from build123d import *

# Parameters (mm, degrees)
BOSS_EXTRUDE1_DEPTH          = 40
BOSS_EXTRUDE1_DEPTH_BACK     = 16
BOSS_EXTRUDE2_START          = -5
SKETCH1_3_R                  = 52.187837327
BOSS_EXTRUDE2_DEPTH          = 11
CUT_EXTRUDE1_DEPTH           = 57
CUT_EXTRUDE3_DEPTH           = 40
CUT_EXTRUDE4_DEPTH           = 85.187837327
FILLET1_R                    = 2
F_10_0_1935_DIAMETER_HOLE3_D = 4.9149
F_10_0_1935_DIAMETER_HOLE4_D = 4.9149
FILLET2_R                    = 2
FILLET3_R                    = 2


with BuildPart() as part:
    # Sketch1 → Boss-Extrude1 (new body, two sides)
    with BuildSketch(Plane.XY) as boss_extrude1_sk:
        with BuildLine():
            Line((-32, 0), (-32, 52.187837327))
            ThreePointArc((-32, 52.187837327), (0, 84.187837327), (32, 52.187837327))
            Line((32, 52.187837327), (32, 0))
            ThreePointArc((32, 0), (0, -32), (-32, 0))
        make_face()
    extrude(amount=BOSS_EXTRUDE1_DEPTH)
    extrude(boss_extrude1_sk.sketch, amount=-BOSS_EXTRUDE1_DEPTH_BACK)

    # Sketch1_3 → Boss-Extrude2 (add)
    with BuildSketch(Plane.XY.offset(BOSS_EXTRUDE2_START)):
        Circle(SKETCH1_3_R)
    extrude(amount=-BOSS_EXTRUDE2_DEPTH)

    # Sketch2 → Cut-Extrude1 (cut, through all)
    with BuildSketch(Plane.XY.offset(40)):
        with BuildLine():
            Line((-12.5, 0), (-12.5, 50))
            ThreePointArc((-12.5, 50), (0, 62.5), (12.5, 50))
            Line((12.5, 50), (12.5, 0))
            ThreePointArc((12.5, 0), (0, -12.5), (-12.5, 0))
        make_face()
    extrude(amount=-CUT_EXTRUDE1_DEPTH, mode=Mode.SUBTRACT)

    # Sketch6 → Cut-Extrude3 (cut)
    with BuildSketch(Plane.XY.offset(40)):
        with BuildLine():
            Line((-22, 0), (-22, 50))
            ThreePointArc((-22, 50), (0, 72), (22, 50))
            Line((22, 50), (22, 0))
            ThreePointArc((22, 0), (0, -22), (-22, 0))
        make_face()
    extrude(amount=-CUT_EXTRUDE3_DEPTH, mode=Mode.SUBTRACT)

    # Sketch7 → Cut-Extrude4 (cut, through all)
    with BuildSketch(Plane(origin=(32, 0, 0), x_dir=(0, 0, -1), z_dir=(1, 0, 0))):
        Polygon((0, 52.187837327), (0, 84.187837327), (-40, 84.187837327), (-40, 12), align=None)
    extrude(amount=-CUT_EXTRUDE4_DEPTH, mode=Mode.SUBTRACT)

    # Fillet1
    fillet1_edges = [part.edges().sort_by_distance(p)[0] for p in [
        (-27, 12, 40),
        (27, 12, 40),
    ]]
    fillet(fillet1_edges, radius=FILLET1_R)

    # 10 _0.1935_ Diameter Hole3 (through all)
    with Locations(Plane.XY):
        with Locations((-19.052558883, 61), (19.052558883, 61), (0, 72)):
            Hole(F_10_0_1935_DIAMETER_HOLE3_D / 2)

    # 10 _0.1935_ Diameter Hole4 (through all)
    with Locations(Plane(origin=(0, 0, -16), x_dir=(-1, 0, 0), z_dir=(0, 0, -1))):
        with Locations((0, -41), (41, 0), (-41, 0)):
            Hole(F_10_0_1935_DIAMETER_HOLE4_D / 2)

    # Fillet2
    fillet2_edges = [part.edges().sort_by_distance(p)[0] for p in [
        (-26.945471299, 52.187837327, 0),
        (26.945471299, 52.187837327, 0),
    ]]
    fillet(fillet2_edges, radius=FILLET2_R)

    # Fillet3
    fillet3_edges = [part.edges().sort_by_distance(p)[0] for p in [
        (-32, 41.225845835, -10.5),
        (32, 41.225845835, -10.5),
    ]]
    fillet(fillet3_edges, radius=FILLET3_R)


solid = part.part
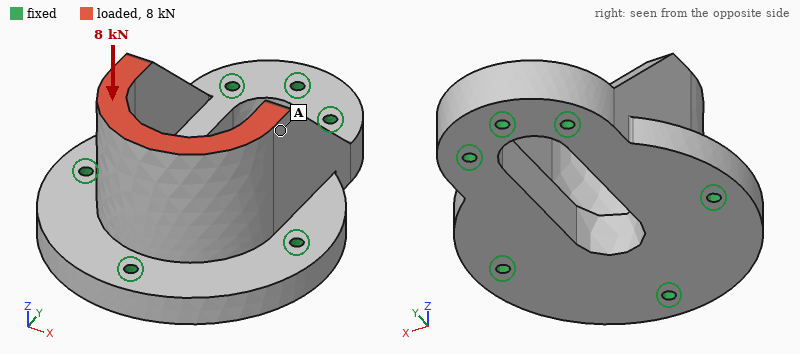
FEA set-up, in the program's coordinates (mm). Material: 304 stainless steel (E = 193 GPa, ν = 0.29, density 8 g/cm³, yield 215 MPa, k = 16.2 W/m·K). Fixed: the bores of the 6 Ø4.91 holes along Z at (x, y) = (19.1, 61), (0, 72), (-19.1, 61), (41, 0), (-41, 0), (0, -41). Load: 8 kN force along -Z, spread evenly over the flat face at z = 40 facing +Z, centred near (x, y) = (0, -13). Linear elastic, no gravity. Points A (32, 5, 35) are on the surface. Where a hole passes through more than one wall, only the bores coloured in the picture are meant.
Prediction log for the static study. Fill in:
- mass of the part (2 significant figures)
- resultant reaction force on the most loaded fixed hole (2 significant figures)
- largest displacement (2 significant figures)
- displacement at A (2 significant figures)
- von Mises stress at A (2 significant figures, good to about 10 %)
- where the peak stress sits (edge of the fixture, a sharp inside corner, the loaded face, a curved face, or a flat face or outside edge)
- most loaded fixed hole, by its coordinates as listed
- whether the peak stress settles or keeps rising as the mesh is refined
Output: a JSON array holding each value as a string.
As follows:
["1.4 kg", "3.4 kN", "6.9 µm", "4.3 µm", "7.1 MPa", "edge of the fixture", "(0, -41)", "keeps rising"]
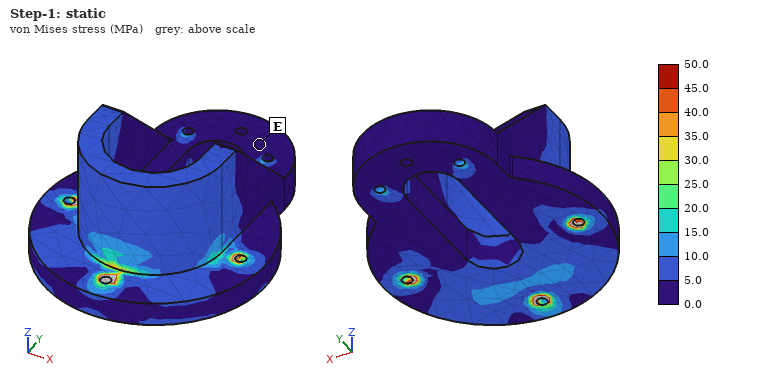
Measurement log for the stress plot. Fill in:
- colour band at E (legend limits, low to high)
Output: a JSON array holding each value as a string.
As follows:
["0.0 to 5.0 MPa"]
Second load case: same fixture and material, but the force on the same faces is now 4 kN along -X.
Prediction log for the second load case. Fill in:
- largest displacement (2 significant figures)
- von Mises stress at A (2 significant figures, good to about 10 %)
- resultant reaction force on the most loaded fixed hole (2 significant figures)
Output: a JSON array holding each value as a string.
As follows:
["22 µm", "20 MPa", "3.2 kN"]
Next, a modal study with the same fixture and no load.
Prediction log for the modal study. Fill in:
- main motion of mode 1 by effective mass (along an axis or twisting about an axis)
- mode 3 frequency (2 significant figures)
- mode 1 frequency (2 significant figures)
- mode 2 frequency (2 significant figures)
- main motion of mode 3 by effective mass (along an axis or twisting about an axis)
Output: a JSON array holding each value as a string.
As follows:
["along X", "8100 Hz", "5700 Hz", "6500 Hz", "along Z"]
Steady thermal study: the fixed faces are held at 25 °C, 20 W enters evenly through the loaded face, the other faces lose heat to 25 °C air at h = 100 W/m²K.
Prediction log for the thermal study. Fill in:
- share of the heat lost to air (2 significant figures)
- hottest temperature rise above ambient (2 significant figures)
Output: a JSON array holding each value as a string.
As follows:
["84 %", "30 K"]
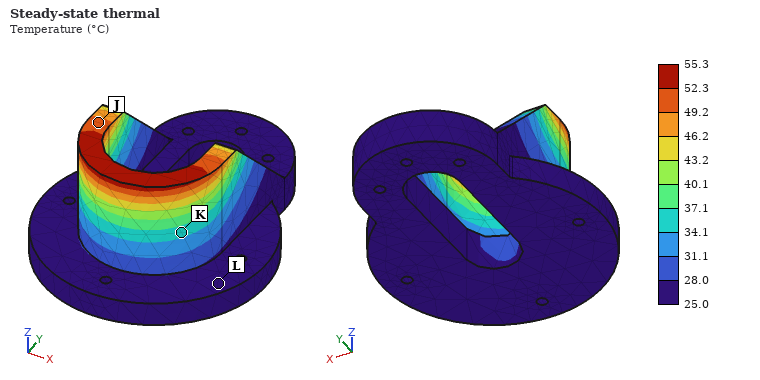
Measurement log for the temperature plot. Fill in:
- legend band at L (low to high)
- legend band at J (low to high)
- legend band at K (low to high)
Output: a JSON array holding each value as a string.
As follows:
["25.0 to 28.0 °C", "49.2 to 52.3 °C", "34.1 to 37.1 °C"]
